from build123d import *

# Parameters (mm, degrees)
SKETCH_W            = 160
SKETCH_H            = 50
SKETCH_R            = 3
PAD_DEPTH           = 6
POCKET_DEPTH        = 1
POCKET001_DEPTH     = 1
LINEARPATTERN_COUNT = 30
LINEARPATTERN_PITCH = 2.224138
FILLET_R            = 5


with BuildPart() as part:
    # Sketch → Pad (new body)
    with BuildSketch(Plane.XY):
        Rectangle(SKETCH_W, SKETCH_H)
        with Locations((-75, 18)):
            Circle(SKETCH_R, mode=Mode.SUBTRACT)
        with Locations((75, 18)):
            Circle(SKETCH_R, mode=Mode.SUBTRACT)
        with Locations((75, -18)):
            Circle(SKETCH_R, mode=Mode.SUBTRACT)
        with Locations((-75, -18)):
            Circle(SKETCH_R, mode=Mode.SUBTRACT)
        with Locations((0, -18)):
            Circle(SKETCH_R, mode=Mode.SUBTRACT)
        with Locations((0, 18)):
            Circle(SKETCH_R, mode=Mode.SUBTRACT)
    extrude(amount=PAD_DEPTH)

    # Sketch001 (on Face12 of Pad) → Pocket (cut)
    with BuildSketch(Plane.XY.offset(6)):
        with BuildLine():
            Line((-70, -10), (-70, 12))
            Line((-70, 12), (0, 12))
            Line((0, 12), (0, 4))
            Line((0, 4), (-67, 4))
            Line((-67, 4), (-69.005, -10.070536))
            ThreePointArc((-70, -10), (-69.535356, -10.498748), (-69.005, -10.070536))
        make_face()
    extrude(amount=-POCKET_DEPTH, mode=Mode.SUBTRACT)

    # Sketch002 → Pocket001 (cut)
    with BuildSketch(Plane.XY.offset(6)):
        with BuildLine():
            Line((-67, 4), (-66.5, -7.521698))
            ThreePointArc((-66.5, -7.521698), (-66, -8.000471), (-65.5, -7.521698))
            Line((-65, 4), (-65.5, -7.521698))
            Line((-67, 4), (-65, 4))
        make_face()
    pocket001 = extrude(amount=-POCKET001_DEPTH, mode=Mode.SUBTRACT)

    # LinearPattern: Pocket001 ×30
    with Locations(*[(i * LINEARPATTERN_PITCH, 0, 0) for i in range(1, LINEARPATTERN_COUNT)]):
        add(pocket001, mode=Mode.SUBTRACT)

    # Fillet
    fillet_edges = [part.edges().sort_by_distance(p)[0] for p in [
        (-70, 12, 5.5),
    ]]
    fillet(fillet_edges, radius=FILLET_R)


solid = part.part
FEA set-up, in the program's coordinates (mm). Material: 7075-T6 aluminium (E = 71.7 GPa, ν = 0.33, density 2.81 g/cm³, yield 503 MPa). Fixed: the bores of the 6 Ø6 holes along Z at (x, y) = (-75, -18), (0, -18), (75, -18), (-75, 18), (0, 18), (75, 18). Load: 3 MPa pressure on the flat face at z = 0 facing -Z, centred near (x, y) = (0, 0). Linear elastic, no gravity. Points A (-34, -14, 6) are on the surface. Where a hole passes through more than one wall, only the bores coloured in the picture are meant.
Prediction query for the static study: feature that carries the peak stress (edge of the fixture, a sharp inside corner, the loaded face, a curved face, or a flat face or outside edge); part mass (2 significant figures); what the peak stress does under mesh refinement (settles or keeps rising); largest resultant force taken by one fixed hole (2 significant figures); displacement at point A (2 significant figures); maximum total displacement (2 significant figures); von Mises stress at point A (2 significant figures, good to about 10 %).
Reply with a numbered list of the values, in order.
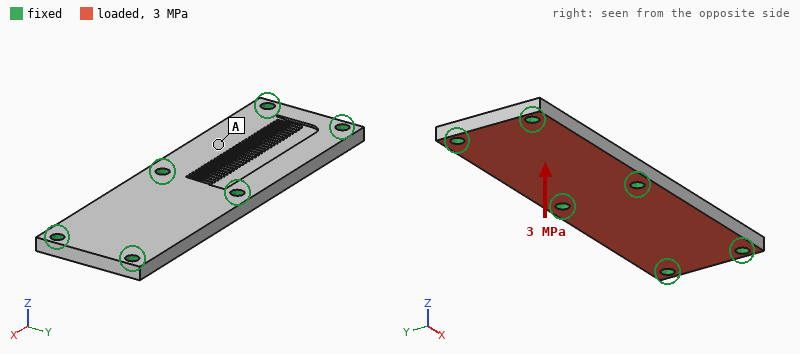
1. edge of the fixture
2. 130 g
3. keeps rising
4. 5.7 kN
5. 0.20 mm
6. 0.22 mm
7. 110 MPa
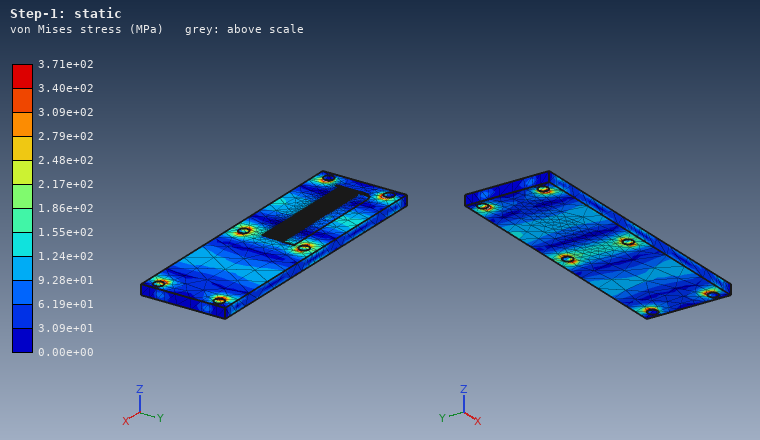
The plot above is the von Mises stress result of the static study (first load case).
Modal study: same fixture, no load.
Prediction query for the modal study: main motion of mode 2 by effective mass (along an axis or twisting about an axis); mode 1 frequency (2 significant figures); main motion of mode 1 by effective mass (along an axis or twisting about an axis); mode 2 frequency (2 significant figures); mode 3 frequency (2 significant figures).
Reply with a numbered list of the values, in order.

1. along Z
2. 5200 Hz
3. twisting about Y
4. 5400 Hz
5. 7400 Hz
